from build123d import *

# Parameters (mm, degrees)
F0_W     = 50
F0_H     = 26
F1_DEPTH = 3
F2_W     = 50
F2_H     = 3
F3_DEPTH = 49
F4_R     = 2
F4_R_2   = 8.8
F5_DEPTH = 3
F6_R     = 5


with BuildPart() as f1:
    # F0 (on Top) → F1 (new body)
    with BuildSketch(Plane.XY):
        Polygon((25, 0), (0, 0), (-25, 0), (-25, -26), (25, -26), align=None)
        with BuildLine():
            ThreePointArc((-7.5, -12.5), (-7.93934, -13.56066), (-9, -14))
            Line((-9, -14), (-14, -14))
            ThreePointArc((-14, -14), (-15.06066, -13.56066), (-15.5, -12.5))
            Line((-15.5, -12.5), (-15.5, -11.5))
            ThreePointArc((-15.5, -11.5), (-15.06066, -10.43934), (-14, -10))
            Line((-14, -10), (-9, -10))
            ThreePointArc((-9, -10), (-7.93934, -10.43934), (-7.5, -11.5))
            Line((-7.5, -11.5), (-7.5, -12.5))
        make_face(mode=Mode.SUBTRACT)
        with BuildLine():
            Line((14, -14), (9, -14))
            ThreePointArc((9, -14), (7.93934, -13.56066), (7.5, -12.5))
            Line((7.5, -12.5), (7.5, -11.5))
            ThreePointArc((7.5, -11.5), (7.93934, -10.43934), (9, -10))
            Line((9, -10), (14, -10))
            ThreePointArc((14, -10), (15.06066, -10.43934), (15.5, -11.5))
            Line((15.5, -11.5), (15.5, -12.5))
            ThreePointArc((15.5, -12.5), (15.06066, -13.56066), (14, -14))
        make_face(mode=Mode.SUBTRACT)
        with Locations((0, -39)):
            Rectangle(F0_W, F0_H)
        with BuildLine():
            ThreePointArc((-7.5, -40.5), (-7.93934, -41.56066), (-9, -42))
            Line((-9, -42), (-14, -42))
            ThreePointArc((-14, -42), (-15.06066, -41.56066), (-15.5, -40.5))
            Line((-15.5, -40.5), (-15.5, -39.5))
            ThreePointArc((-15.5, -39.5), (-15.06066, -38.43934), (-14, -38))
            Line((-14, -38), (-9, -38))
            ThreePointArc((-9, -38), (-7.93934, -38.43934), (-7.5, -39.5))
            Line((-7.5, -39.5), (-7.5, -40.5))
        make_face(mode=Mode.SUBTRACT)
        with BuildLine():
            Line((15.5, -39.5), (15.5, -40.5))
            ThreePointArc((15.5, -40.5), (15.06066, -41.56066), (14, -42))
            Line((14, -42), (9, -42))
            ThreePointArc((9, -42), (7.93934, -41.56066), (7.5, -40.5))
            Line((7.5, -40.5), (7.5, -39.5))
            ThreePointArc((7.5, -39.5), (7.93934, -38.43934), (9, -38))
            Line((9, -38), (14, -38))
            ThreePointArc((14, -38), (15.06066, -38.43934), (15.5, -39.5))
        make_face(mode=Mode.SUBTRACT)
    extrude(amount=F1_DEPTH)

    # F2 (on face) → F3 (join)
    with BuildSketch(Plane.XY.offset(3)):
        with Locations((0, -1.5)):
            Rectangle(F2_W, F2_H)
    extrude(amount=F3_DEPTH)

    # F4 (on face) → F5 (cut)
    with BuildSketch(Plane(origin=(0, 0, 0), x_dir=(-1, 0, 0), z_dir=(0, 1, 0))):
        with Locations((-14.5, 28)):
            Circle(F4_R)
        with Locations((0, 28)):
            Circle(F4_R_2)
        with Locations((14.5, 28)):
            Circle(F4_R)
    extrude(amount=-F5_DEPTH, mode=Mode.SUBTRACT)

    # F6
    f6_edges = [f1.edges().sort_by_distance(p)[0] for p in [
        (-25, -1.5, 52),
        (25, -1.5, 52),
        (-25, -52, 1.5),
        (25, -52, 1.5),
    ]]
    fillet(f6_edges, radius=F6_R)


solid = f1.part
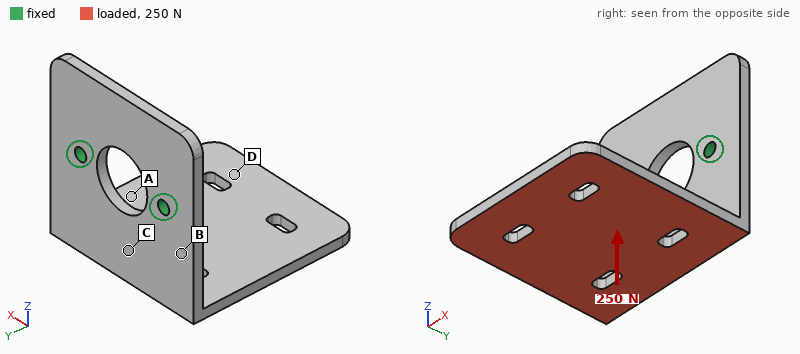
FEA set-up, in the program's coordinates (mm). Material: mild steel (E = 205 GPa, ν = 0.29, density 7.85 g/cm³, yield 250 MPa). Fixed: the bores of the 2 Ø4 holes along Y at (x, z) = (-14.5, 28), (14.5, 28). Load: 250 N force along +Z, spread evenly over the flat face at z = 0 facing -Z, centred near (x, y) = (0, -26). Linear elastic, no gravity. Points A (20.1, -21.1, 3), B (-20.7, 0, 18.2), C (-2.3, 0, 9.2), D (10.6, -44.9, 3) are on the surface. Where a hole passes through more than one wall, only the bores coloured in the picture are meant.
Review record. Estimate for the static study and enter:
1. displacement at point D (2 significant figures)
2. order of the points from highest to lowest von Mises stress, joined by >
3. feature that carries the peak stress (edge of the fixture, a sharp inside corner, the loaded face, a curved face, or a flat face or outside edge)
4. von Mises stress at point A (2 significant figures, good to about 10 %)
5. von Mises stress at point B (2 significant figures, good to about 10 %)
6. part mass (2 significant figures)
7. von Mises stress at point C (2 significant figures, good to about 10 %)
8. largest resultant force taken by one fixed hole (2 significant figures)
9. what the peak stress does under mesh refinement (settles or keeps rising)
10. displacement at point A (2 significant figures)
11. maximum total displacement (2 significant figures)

0.49 mm
B > C > A > D
edge of the fixture
31 MPa
94 MPa
110 g
66 MPa
130 N
keeps rising
0.21 mm
0.58 mm
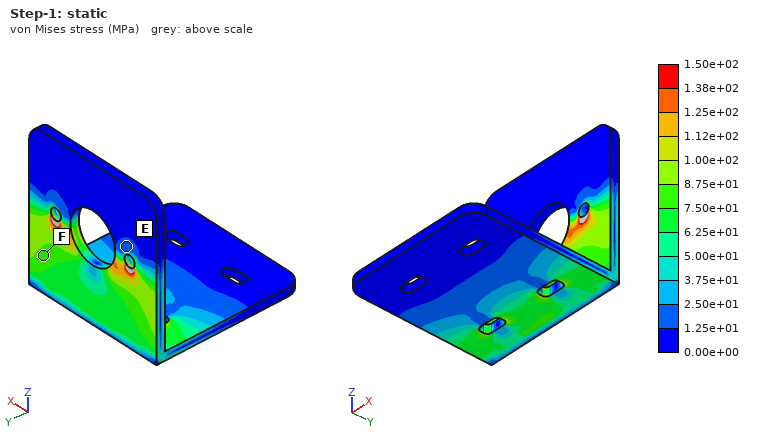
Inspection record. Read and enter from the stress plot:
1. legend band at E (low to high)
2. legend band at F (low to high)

1.25e+01 to 2.50e+01 MPa
7.50e+01 to 8.75e+01 MPa
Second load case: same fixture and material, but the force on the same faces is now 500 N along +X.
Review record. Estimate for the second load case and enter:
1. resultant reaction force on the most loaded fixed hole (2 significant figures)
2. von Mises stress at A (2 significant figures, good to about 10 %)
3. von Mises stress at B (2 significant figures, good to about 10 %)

580 N
21 MPa
72 MPa
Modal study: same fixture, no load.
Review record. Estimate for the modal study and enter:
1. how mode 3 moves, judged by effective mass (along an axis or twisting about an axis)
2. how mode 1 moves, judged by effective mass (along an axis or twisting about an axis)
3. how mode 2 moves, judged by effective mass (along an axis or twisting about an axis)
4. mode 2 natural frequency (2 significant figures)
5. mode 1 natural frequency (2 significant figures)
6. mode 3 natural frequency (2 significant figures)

along Y
along Z
along X
1100 Hz
500 Hz
1700 Hz
